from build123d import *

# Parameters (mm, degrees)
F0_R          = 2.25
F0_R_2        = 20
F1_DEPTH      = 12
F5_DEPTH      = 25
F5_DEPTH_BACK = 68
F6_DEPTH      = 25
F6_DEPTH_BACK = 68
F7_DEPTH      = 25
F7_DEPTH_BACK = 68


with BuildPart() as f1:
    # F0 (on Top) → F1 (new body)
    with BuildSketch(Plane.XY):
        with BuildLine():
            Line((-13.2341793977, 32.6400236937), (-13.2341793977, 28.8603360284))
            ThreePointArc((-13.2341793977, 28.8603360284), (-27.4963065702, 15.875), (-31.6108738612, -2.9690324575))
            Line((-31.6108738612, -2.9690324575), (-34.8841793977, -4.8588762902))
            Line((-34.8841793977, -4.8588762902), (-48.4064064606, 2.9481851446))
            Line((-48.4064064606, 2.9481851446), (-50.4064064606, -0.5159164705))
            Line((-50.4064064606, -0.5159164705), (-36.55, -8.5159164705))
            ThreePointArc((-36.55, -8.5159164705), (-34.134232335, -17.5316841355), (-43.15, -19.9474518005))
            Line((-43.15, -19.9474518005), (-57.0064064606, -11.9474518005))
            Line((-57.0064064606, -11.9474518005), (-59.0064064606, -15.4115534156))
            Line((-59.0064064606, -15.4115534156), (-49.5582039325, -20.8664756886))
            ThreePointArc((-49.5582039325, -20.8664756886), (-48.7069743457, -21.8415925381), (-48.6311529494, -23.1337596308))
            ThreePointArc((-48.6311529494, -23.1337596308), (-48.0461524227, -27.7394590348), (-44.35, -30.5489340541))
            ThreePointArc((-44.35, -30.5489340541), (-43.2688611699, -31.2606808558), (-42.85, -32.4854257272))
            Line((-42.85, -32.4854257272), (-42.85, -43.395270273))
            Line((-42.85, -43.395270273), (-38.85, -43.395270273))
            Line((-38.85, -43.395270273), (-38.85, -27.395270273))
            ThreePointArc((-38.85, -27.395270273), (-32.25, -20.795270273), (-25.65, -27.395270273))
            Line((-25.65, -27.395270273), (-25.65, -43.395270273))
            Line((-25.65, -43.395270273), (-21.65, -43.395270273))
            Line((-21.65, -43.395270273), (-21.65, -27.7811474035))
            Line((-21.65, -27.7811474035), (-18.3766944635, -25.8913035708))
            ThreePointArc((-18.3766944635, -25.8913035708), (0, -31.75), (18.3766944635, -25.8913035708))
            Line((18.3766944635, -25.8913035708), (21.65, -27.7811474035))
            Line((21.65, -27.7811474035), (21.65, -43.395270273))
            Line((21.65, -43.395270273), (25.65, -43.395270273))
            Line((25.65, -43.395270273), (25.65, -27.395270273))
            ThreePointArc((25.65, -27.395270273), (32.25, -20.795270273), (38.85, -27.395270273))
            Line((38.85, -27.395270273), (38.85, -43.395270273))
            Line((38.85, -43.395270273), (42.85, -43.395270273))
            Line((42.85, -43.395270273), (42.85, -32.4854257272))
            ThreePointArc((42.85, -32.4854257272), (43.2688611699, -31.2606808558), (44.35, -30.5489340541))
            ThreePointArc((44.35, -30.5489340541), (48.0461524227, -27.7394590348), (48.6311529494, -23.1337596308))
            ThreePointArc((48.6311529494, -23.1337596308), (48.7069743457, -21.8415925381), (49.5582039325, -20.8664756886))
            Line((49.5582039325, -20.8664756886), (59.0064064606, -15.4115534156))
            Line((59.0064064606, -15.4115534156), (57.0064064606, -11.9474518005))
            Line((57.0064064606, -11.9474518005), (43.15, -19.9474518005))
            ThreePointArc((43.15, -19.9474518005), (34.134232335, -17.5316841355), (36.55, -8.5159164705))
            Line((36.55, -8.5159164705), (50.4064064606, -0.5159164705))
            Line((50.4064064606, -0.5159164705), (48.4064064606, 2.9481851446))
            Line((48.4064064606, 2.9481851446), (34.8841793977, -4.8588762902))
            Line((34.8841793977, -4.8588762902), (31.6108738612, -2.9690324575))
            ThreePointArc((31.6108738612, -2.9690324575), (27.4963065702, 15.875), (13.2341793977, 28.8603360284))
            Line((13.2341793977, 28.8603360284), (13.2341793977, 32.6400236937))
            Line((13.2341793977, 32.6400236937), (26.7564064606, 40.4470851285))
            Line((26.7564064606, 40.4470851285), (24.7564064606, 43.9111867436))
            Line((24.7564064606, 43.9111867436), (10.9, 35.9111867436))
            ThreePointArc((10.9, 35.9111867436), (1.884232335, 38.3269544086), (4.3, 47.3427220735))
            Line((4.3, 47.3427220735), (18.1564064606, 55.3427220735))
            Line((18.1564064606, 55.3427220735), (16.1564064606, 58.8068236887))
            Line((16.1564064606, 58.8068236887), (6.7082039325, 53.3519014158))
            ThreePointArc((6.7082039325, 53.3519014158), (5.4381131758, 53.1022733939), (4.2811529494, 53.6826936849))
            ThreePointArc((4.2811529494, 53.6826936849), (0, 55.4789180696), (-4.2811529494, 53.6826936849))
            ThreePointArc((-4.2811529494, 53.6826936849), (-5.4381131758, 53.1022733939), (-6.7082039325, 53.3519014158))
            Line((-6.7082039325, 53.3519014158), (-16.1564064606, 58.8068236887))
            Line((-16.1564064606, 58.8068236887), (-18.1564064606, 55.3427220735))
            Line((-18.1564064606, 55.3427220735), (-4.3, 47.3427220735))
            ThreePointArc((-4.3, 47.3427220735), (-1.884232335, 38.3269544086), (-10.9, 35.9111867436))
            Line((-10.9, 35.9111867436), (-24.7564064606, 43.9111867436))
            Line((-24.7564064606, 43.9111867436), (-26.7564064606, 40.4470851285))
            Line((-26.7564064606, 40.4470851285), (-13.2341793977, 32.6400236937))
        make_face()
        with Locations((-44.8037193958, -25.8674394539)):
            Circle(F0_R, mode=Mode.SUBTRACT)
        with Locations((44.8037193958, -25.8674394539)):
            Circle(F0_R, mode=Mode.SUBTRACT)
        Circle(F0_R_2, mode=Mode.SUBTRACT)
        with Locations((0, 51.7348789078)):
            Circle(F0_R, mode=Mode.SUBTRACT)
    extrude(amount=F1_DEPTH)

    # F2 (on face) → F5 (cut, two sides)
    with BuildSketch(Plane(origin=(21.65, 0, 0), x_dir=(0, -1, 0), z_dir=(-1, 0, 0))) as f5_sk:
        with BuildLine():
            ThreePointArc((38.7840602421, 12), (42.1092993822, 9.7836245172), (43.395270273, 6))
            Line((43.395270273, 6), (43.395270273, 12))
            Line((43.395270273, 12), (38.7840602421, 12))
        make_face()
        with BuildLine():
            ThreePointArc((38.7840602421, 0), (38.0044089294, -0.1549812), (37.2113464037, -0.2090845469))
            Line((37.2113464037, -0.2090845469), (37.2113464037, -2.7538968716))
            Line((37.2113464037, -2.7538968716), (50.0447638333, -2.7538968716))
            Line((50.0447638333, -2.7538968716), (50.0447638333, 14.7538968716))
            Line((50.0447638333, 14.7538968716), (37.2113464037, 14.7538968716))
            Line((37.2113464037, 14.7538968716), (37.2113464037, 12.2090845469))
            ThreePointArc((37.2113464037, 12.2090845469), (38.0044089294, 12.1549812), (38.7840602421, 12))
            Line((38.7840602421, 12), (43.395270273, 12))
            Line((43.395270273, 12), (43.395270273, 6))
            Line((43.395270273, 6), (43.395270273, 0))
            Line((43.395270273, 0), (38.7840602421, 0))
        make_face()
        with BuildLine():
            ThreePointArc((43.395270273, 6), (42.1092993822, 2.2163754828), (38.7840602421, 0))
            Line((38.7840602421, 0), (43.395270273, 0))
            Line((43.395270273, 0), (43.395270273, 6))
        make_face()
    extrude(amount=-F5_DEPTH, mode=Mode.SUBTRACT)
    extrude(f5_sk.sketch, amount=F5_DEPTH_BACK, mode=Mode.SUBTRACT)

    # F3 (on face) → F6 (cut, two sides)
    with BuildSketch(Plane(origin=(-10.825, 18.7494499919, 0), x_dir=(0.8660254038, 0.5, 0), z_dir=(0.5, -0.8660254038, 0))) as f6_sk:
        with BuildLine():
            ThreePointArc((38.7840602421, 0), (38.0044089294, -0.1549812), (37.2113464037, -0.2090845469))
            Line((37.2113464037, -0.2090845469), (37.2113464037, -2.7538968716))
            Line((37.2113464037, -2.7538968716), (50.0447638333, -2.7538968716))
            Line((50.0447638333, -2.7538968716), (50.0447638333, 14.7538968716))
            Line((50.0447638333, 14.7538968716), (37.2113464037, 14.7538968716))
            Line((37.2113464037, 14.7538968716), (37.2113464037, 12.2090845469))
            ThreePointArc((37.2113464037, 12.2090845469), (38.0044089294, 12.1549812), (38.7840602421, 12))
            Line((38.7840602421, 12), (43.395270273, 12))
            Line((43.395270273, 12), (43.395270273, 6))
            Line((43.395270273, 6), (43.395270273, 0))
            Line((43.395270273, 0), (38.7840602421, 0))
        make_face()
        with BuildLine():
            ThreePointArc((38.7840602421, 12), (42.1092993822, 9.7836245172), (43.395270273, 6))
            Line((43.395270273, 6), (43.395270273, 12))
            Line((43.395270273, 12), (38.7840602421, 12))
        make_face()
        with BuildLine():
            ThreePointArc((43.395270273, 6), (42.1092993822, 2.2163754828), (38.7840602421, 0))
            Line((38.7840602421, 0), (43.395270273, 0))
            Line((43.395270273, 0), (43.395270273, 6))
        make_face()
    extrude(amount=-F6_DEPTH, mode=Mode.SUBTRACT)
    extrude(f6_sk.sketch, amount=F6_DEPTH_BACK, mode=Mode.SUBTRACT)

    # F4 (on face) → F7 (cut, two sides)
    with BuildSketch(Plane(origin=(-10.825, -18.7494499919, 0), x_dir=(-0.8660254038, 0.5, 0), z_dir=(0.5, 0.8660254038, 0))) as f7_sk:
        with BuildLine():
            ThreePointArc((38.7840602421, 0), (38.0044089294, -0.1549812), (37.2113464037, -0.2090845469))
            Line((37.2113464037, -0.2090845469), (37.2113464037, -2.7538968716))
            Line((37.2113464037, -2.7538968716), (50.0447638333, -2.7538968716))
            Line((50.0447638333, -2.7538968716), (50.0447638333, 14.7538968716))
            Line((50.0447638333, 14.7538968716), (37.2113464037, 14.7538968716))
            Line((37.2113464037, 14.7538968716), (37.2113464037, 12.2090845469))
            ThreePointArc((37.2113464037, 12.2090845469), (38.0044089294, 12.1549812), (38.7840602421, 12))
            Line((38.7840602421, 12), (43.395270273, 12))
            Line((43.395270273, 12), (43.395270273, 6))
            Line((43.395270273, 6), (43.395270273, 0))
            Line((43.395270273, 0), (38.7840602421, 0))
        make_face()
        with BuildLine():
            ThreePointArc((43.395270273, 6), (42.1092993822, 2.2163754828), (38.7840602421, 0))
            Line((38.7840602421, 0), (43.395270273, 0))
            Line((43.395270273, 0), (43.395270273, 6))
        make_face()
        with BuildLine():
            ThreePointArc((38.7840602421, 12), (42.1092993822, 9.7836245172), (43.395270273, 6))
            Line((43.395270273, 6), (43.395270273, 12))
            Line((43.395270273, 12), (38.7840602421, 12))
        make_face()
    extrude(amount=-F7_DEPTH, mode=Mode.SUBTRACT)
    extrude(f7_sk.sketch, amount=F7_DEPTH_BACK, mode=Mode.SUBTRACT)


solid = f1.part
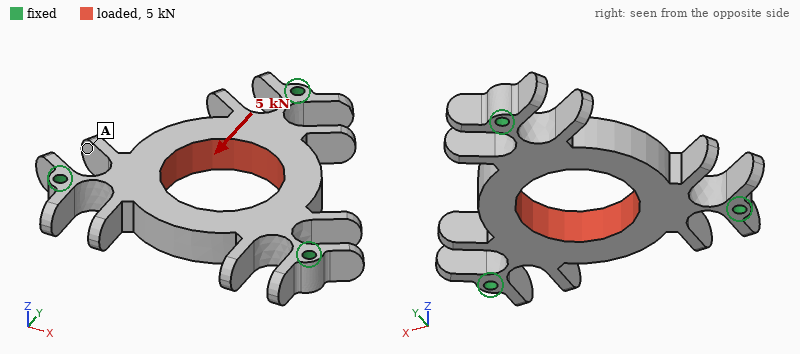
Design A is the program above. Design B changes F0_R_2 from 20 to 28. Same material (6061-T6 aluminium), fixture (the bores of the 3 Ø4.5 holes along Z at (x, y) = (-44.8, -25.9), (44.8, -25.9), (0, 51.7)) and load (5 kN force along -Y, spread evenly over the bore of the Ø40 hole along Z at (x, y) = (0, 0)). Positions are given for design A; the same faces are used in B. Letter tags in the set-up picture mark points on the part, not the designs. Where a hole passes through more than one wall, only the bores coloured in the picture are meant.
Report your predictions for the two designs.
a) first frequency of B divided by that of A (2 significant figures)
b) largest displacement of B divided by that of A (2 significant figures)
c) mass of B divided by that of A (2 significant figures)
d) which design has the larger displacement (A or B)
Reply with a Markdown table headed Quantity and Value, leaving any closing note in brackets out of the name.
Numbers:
| Quantity | Value |
|---|---|
| first frequency of B divided by that of A | 0.79 |
| largest displacement of B divided by that of A | 5.4 |
| mass of B divided by that of A | 0.63 |
| which design has the larger displacement | B |
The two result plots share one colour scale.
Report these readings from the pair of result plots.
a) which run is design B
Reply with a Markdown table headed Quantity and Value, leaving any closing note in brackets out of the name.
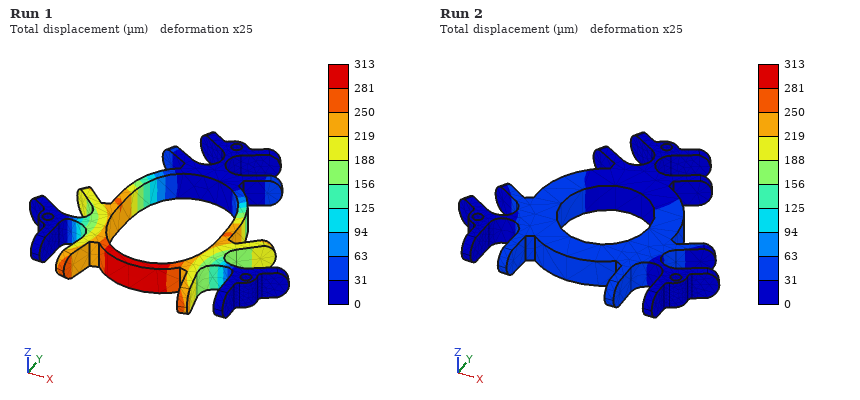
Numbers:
| Quantity | Value |
|---|---|
| which run is design B | Run 1 |
